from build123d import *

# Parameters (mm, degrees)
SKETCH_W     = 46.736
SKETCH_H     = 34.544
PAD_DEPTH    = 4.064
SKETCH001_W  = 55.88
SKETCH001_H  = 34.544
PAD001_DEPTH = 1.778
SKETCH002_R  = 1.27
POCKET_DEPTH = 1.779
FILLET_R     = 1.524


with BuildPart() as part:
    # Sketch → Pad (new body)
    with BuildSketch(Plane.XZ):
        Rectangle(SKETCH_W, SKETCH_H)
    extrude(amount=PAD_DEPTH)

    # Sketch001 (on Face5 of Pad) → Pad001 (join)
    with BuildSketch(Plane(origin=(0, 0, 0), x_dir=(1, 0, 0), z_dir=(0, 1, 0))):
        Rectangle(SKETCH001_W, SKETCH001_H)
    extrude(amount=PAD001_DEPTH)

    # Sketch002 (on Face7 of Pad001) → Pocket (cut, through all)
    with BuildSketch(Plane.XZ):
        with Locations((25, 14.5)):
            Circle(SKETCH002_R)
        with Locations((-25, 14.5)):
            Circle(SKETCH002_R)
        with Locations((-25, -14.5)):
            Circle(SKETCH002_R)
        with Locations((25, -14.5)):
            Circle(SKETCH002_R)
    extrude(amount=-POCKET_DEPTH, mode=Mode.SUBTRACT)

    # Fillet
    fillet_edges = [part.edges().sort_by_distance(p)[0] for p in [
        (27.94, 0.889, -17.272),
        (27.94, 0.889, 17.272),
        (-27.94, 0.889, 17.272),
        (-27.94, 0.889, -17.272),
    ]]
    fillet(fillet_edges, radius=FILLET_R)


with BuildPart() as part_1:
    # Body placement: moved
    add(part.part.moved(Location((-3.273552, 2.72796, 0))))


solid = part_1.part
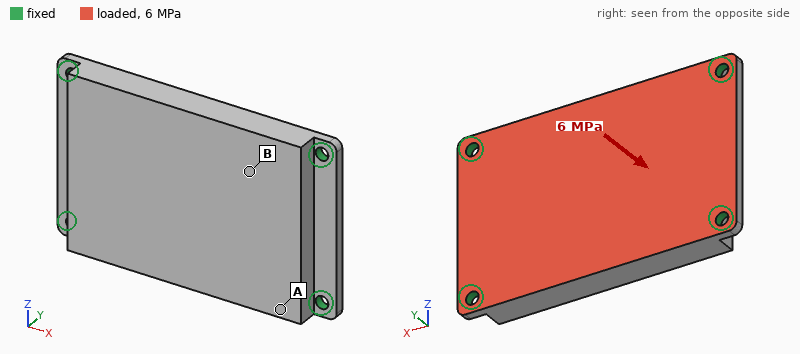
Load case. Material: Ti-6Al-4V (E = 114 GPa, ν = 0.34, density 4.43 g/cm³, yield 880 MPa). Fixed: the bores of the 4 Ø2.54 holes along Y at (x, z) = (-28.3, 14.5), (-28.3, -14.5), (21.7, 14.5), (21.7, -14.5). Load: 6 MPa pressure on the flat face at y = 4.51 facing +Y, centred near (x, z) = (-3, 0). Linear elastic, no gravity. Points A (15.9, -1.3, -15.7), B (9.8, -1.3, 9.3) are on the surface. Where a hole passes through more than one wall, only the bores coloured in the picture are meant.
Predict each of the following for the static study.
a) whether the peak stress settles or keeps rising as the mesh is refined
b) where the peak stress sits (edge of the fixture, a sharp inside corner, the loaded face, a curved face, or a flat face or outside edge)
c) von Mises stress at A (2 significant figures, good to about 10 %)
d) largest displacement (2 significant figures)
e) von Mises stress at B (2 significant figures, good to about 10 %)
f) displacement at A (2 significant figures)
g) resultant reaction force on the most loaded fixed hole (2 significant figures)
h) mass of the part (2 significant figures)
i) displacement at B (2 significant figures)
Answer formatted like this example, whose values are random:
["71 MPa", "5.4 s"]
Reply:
["keeps rising", "edge of the fixture", "85 MPa", "0.15 mm", "160 MPa", "0.056 mm", "4.7 kN", "44 g", "0.11 mm"]
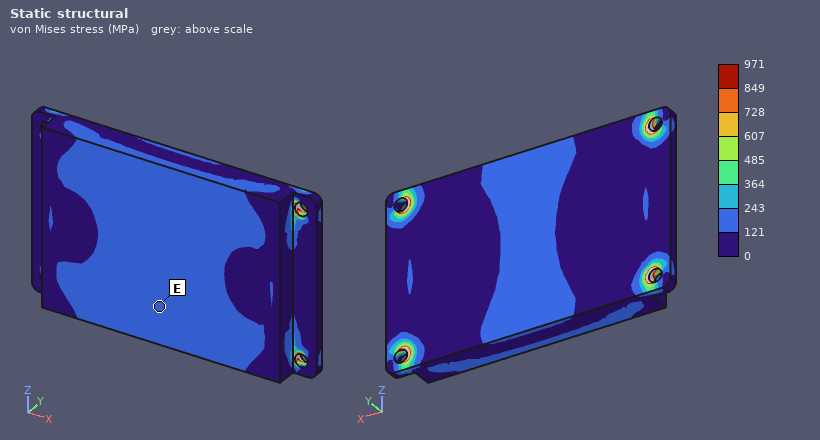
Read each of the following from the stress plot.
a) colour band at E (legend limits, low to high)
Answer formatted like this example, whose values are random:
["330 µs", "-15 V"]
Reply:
["121 to 243 MPa"]
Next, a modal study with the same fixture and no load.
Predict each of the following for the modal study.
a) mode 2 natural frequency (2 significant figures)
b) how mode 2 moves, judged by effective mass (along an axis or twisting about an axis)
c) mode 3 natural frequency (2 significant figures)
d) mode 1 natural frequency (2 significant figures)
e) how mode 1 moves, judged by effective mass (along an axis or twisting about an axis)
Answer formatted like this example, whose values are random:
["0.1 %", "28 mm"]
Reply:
["12 kHz", "twisting about X", "16 kHz", "7000 Hz", "along Y"]
